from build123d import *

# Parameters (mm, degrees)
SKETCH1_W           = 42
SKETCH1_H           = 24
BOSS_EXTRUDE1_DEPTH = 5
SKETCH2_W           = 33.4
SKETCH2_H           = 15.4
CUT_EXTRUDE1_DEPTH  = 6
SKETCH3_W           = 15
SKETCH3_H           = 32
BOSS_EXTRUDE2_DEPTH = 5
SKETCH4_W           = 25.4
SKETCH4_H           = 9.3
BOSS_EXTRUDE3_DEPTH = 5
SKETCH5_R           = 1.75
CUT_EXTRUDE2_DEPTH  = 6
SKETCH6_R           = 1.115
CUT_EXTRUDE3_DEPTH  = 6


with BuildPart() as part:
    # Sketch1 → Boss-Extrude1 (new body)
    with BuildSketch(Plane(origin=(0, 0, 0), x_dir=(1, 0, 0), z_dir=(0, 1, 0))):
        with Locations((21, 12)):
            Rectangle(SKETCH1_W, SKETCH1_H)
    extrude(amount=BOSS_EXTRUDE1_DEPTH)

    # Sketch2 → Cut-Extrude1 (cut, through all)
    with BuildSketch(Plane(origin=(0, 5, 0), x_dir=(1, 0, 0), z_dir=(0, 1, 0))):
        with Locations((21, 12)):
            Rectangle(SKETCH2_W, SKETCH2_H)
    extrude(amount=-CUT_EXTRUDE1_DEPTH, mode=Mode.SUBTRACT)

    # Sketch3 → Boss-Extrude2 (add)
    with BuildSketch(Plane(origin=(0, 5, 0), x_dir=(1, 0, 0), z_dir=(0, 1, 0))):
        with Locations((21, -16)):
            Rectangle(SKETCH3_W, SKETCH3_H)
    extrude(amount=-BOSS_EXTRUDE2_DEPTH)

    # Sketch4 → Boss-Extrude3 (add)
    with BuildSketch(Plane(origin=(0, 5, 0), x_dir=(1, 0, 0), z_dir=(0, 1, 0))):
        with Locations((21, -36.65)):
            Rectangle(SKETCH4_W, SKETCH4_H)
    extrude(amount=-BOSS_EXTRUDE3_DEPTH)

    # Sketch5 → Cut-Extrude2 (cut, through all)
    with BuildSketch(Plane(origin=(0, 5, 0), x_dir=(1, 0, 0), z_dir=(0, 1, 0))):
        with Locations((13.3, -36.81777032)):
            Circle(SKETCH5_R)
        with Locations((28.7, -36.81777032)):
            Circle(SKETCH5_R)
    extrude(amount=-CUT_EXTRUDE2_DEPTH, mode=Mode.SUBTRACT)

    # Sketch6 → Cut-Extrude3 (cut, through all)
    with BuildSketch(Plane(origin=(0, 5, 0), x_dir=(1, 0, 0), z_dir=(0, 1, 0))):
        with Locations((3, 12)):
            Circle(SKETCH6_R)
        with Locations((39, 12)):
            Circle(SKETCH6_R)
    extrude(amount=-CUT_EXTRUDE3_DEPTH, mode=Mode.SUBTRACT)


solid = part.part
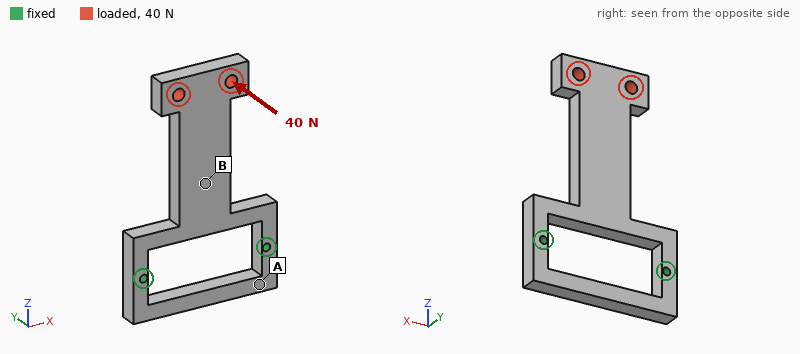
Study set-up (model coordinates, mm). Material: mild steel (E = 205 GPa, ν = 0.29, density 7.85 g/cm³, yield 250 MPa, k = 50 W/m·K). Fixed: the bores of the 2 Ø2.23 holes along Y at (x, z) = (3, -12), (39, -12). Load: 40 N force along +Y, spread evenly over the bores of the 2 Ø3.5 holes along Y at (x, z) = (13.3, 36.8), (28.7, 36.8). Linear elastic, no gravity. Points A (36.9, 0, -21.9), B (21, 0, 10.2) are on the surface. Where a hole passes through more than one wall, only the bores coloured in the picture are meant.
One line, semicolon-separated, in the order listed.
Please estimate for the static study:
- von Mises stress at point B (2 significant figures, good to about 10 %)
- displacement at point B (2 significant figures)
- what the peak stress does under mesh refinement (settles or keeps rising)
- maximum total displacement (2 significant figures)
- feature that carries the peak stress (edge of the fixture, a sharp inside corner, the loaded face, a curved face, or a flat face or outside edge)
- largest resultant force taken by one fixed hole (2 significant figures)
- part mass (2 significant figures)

18 MPa; 0.041 mm; keeps rising; 0.14 mm; edge of the fixture; 20 N; 46 g
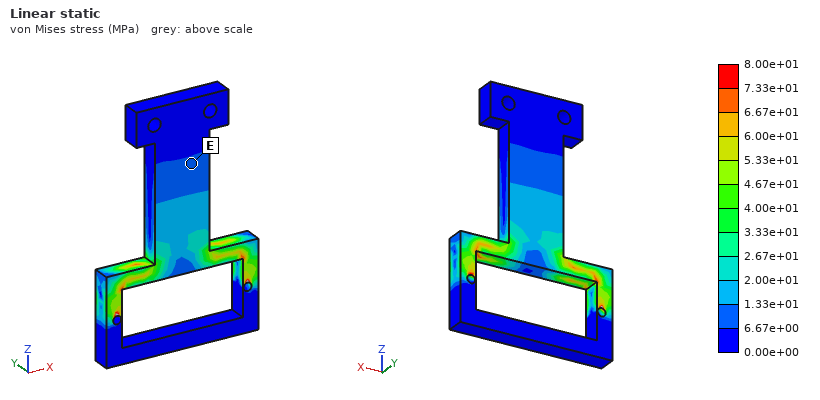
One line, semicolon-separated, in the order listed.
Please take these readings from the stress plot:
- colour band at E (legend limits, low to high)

6.67e+00 to 1.33e+01 MPa
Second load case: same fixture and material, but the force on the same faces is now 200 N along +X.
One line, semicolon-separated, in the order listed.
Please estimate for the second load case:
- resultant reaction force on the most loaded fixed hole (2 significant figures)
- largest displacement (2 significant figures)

280 N; 60 µm
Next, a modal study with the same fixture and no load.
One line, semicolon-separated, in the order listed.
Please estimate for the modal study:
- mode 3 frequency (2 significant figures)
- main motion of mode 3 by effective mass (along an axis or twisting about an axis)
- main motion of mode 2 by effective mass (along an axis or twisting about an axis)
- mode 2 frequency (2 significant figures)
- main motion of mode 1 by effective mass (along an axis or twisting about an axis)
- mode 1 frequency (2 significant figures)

5800 Hz; along Z; along X; 2700 Hz; along Y; 760 Hz
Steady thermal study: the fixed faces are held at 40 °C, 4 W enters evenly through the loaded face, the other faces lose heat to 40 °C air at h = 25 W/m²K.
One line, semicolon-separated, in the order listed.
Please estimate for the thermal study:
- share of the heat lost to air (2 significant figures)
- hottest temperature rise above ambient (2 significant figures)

51 %; 48 K
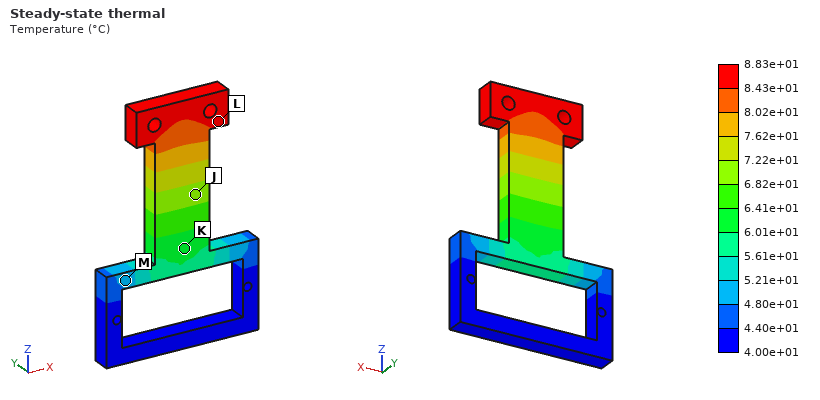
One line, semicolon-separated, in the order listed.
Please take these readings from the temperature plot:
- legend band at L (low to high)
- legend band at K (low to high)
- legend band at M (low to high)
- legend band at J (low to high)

8.43e+01 to 8.83e+01 °C; 6.01e+01 to 6.41e+01 °C; 4.80e+01 to 5.21e+01 °C; 6.82e+01 to 7.22e+01 °C
